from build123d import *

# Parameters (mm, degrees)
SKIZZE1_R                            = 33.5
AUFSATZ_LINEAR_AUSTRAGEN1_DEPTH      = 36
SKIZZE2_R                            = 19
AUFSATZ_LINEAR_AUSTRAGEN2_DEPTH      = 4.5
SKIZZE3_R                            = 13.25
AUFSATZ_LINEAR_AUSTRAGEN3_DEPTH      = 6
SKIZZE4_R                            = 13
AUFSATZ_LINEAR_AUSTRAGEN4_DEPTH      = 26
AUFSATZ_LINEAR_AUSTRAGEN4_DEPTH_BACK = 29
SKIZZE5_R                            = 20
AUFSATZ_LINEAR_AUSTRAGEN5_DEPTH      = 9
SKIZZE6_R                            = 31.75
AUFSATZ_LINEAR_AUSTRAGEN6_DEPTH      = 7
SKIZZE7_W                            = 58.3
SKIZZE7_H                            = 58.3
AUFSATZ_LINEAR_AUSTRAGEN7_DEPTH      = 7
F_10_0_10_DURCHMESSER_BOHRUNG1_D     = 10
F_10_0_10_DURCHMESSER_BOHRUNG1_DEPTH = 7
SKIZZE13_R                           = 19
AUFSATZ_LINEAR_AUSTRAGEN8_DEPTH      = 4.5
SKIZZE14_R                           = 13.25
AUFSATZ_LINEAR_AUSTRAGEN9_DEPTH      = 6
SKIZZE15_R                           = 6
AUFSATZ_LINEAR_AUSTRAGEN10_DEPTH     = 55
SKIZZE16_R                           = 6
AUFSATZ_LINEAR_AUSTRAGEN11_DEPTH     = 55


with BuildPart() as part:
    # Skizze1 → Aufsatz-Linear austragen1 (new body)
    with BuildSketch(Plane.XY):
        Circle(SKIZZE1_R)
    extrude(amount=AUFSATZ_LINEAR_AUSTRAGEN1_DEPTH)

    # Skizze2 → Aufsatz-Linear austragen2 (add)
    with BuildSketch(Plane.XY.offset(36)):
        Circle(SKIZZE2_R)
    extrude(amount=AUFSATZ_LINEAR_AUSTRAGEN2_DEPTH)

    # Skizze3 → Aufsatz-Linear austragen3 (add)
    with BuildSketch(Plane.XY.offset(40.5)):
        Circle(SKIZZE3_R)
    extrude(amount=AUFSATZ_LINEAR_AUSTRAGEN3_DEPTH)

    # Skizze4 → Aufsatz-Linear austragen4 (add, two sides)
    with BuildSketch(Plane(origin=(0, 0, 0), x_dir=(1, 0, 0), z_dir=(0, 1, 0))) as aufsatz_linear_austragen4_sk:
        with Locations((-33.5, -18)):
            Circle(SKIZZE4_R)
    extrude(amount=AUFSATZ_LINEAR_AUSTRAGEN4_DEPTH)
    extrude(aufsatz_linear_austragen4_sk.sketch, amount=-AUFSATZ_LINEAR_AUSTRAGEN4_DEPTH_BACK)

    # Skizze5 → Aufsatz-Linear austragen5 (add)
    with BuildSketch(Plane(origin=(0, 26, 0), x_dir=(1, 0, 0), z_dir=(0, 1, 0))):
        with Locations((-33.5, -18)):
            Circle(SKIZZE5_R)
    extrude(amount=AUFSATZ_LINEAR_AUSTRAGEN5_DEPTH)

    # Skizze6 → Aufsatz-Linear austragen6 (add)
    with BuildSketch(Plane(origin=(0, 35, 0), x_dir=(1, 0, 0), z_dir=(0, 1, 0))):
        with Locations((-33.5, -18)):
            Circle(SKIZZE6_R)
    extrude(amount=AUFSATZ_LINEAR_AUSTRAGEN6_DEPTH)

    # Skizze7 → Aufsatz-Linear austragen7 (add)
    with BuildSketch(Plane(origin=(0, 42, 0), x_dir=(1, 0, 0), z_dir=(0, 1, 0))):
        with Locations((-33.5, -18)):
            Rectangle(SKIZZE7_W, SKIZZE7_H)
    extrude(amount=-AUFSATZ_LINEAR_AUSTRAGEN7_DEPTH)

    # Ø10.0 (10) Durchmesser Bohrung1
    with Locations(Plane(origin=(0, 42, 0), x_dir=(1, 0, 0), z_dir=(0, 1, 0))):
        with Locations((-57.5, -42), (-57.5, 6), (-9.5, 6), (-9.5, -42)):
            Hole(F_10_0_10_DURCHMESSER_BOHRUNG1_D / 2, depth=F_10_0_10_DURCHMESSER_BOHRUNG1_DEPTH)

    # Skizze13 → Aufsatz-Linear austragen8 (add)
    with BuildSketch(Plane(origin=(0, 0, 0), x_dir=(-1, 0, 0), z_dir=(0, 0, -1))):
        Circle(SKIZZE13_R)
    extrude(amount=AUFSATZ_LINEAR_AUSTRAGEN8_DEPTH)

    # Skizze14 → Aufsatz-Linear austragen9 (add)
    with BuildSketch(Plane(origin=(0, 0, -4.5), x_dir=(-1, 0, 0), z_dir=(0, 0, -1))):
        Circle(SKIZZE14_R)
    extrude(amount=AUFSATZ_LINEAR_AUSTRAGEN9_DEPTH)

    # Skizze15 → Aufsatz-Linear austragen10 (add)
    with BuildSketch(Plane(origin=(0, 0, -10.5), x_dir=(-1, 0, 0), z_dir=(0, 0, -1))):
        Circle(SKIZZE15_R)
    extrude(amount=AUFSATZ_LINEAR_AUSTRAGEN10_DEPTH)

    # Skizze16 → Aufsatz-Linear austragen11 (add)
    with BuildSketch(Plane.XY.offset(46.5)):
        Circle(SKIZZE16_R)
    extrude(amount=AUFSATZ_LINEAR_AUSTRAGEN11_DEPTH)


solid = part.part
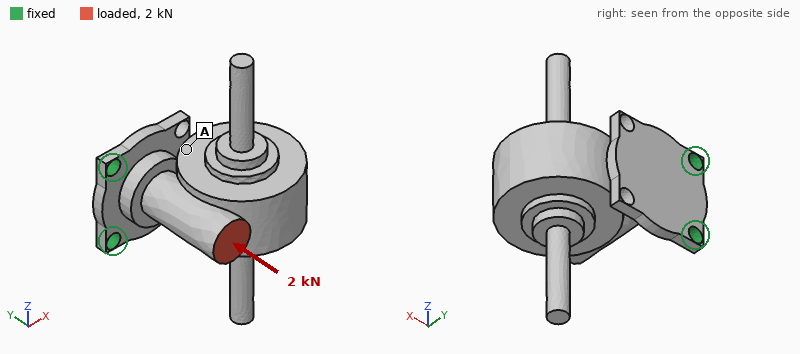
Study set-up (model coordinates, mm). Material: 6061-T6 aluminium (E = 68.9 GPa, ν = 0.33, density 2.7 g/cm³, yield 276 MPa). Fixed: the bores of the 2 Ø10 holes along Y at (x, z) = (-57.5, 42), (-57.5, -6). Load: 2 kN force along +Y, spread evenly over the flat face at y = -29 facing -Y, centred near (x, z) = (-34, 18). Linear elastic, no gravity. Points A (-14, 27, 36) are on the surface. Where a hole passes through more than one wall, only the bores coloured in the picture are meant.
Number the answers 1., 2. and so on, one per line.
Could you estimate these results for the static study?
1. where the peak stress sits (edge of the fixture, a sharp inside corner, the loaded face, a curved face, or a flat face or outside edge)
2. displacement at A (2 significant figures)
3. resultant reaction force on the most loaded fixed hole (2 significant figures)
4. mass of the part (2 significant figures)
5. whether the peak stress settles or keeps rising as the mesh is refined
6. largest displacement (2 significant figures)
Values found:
1. edge of the fixture
2. 0.14 mm
3. 1.0 kN
4. 570 g
5. keeps rising
6. 0.34 mm
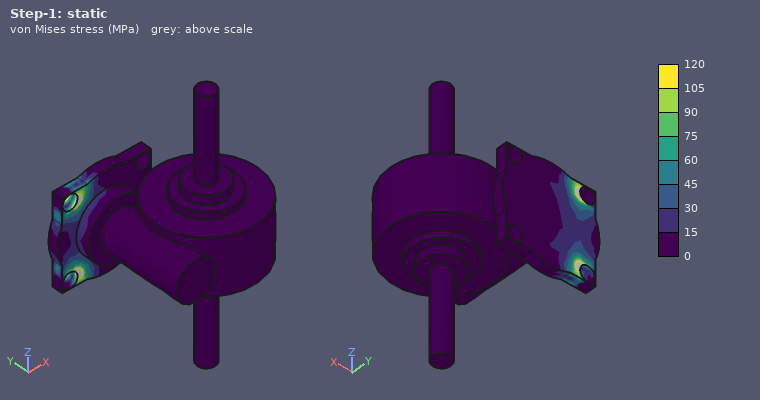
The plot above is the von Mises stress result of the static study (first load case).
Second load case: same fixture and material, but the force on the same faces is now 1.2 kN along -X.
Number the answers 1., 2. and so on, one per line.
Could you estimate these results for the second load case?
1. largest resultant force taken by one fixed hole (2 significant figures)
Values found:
1. 670 N
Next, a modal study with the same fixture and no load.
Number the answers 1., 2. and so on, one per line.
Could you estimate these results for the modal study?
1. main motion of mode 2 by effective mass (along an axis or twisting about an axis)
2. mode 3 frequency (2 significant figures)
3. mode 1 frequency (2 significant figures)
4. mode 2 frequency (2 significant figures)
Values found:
1. along Z
2. 2000 Hz
3. 340 Hz
4. 1000 Hz
